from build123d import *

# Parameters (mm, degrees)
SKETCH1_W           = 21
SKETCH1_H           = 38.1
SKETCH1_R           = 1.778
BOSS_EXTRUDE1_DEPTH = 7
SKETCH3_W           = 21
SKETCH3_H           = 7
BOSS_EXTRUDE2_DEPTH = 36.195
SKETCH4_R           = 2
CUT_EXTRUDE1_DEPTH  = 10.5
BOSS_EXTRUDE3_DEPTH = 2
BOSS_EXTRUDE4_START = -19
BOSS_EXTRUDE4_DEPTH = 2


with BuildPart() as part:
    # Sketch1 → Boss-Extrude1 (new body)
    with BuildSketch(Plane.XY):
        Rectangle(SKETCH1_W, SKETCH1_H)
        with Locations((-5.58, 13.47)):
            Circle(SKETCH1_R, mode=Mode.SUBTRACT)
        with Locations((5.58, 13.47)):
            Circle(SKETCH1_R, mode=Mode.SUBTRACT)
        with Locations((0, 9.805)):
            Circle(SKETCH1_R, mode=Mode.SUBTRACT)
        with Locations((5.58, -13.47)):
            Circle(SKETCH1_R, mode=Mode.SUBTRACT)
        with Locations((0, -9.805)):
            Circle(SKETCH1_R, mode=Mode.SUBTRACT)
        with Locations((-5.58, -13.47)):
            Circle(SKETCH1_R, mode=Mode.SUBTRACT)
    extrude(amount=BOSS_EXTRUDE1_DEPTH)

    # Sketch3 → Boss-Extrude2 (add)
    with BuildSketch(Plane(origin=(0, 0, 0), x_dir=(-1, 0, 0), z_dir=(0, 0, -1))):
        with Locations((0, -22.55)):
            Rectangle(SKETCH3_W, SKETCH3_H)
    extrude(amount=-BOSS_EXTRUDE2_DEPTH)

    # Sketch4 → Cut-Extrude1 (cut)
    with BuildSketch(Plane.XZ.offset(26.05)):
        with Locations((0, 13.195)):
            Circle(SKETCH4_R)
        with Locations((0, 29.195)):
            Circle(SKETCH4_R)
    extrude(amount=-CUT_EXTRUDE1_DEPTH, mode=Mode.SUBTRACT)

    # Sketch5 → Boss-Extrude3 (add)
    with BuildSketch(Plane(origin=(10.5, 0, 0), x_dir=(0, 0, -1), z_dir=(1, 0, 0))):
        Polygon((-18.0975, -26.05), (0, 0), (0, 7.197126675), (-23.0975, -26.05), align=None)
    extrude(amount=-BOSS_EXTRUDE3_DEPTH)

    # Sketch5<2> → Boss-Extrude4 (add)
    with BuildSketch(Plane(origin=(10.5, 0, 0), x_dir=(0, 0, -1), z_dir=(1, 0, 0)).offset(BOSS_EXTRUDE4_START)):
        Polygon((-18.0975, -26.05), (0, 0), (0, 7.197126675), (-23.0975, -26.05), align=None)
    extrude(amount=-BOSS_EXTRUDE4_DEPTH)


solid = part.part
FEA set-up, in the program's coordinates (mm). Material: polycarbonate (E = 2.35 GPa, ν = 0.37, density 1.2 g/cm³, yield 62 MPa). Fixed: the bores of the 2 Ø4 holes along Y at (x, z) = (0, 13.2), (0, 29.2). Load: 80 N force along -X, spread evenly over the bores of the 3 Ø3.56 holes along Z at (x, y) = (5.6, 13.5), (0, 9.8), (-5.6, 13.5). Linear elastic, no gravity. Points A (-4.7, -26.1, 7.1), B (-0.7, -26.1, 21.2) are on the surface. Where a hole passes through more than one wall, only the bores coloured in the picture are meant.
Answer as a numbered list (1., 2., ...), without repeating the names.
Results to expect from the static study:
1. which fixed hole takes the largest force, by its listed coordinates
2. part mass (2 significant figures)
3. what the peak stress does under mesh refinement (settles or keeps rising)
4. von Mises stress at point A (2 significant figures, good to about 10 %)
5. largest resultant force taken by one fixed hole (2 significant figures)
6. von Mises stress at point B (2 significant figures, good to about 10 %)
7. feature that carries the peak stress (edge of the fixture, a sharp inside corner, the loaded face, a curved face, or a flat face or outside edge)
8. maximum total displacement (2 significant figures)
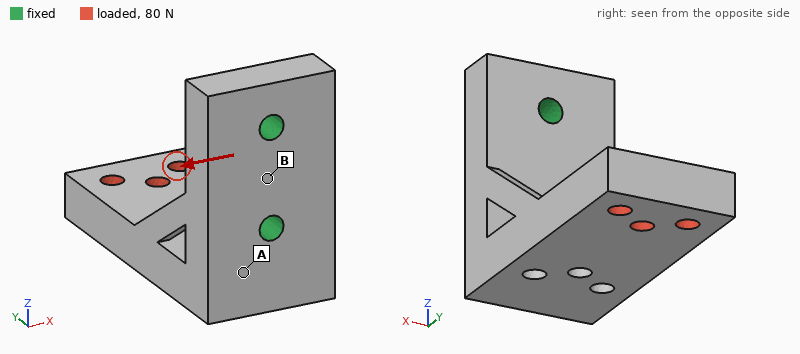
1. (0, 13.2)
2. 13 g
3. keeps rising
4. 5.8 MPa
5. 110 N
6. 2.6 MPa
7. edge of the fixture
8. 0.63 mm
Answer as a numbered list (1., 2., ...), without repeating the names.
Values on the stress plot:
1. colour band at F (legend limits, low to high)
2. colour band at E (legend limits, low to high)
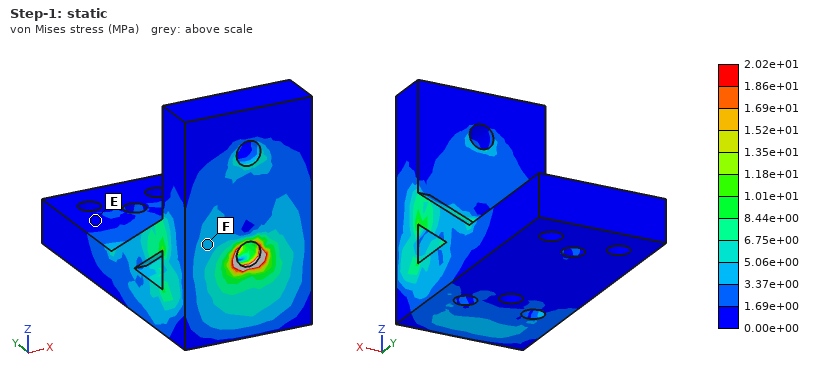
1. 3.37e+00 to 5.06e+00 MPa
2. 0.00e+00 to 1.69e+00 MPa
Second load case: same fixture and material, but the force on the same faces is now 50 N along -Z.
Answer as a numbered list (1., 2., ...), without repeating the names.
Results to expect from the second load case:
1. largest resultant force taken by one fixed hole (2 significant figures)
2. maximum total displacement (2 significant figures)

1. 59 N
2. 0.62 mm
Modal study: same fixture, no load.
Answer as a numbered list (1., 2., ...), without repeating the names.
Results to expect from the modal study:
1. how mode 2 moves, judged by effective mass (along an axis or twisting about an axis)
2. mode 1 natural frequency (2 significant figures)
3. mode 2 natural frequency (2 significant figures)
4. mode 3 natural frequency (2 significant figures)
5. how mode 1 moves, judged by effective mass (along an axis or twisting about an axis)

1. along X
2. 950 Hz
3. 1100 Hz
4. 3200 Hz
5. along Z
